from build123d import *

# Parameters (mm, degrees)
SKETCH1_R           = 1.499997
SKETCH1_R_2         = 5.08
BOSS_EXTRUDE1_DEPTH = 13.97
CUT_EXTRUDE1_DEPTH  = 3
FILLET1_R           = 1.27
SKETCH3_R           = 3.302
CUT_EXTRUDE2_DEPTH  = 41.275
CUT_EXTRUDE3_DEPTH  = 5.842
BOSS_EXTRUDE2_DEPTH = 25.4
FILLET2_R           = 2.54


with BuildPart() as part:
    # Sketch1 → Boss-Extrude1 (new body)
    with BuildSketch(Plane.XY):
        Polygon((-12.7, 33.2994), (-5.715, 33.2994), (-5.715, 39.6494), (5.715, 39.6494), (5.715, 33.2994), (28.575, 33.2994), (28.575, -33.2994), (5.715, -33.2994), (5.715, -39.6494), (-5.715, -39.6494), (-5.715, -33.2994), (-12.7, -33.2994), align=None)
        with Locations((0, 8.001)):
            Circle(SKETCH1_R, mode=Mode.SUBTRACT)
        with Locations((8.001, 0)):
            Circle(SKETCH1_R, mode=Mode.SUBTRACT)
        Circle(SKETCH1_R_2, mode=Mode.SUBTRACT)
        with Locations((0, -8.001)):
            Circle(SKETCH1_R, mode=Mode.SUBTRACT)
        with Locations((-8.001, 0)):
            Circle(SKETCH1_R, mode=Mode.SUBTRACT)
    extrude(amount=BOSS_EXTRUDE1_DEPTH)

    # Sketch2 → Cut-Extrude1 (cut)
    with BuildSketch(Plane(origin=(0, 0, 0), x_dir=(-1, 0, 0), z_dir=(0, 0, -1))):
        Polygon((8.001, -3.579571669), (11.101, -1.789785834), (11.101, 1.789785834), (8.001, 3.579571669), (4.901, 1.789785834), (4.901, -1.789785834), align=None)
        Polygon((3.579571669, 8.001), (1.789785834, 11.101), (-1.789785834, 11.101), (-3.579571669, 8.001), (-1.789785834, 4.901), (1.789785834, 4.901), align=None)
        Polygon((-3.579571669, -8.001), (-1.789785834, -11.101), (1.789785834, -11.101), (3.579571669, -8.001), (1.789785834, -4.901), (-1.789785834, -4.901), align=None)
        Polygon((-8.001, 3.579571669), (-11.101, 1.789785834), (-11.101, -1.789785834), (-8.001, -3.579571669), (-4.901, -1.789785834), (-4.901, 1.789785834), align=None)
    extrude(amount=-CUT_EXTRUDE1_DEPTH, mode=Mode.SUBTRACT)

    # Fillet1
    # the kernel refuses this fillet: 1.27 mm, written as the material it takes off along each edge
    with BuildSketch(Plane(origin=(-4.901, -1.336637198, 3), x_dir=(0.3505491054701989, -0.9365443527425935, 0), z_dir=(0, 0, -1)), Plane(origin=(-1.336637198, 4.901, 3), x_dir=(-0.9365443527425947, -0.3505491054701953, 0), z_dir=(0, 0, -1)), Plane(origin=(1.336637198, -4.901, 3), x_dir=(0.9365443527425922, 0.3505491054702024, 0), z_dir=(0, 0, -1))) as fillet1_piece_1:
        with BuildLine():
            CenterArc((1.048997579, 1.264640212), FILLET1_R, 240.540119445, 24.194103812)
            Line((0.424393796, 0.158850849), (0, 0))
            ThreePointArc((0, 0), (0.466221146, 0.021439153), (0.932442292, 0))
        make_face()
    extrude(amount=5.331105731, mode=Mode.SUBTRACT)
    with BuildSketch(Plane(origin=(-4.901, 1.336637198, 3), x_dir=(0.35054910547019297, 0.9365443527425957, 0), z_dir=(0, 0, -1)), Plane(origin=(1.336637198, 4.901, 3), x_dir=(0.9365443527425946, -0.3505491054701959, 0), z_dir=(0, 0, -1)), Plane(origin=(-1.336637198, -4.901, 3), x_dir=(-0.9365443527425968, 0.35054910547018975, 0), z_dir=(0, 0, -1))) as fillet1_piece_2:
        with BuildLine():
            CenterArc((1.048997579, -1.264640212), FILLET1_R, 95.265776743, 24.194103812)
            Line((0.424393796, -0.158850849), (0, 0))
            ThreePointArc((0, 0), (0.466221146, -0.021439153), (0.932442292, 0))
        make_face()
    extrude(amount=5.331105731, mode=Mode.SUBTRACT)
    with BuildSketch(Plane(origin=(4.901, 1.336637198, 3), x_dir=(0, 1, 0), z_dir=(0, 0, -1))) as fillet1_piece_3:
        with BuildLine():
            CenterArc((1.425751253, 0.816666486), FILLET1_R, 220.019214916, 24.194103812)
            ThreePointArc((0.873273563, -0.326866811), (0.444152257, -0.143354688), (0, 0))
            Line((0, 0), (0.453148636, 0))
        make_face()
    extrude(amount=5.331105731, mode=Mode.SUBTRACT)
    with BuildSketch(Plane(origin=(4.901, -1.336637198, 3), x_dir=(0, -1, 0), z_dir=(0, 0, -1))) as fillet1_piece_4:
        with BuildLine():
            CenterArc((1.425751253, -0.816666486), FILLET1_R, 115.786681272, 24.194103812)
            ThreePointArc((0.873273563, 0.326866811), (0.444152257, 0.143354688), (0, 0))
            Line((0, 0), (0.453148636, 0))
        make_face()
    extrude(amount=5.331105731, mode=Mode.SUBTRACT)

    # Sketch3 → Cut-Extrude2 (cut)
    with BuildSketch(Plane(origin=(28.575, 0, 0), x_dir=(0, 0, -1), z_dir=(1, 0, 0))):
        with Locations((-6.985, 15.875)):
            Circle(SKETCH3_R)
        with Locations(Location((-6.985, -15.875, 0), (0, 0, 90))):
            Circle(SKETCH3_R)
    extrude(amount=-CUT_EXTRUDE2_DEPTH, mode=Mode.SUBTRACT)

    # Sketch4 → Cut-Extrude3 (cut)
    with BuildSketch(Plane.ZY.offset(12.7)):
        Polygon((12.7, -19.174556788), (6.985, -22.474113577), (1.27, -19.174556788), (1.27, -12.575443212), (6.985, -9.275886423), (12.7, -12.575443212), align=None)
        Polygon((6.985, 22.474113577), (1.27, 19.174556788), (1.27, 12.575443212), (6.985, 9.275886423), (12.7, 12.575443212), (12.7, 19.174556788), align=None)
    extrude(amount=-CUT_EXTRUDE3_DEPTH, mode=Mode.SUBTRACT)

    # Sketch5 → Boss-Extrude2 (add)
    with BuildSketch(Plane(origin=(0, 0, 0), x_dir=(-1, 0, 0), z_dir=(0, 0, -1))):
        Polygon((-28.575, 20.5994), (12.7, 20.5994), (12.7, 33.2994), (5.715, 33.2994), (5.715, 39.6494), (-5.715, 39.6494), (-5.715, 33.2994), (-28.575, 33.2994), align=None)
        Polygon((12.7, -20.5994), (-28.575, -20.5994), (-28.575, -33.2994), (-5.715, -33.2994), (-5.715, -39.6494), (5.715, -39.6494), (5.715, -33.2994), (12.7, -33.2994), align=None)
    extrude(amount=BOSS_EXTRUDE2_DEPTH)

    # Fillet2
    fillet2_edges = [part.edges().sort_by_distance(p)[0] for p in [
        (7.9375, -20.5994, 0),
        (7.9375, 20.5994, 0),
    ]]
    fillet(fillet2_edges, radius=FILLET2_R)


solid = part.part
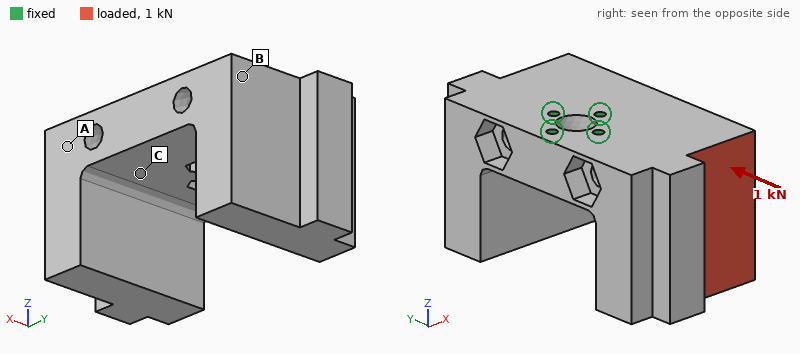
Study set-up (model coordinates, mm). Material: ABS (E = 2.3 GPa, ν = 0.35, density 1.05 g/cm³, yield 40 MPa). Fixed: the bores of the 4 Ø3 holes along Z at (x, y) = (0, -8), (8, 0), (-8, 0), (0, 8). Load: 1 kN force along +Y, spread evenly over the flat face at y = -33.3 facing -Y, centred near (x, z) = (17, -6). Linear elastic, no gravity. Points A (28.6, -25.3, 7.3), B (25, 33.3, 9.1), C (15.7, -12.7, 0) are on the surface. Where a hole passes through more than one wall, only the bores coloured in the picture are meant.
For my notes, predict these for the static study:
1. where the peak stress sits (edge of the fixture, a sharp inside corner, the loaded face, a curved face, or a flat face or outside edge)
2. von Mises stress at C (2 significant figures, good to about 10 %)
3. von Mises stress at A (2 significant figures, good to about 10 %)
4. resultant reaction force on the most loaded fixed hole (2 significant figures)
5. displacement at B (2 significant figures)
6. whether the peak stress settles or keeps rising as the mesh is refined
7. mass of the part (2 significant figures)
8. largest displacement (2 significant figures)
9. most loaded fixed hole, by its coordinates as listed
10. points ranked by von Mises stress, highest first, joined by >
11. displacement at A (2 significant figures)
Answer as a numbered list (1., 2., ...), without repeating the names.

1. edge of the fixture
2. 13 MPa
3. 5.2 MPa
4. 1.0 kN
5. 0.15 mm
6. keeps rising
7. 69 g
8. 0.98 mm
9. (8, 0)
10. C > A > B
11. 0.31 mm
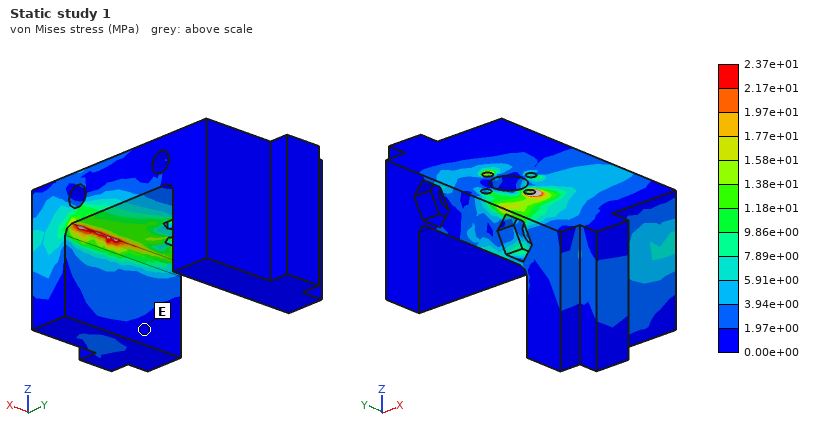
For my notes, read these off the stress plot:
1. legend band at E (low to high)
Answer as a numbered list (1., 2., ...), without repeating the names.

1. 0.00e+00 to 1.97e+00 MPa
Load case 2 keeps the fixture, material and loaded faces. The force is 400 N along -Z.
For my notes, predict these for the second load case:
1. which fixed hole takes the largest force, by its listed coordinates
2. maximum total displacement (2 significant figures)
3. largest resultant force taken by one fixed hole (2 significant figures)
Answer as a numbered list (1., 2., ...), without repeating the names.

1. (0, -8)
2. 0.70 mm
3. 460 N
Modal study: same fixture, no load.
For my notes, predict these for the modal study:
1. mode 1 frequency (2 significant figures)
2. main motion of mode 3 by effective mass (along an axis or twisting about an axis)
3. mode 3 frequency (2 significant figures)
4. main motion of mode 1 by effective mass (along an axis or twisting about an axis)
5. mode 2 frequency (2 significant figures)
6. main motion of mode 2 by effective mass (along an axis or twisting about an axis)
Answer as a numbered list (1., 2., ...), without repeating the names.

1. 960 Hz
2. along X
3. 1200 Hz
4. along Y
5. 1200 Hz
6. along Z
